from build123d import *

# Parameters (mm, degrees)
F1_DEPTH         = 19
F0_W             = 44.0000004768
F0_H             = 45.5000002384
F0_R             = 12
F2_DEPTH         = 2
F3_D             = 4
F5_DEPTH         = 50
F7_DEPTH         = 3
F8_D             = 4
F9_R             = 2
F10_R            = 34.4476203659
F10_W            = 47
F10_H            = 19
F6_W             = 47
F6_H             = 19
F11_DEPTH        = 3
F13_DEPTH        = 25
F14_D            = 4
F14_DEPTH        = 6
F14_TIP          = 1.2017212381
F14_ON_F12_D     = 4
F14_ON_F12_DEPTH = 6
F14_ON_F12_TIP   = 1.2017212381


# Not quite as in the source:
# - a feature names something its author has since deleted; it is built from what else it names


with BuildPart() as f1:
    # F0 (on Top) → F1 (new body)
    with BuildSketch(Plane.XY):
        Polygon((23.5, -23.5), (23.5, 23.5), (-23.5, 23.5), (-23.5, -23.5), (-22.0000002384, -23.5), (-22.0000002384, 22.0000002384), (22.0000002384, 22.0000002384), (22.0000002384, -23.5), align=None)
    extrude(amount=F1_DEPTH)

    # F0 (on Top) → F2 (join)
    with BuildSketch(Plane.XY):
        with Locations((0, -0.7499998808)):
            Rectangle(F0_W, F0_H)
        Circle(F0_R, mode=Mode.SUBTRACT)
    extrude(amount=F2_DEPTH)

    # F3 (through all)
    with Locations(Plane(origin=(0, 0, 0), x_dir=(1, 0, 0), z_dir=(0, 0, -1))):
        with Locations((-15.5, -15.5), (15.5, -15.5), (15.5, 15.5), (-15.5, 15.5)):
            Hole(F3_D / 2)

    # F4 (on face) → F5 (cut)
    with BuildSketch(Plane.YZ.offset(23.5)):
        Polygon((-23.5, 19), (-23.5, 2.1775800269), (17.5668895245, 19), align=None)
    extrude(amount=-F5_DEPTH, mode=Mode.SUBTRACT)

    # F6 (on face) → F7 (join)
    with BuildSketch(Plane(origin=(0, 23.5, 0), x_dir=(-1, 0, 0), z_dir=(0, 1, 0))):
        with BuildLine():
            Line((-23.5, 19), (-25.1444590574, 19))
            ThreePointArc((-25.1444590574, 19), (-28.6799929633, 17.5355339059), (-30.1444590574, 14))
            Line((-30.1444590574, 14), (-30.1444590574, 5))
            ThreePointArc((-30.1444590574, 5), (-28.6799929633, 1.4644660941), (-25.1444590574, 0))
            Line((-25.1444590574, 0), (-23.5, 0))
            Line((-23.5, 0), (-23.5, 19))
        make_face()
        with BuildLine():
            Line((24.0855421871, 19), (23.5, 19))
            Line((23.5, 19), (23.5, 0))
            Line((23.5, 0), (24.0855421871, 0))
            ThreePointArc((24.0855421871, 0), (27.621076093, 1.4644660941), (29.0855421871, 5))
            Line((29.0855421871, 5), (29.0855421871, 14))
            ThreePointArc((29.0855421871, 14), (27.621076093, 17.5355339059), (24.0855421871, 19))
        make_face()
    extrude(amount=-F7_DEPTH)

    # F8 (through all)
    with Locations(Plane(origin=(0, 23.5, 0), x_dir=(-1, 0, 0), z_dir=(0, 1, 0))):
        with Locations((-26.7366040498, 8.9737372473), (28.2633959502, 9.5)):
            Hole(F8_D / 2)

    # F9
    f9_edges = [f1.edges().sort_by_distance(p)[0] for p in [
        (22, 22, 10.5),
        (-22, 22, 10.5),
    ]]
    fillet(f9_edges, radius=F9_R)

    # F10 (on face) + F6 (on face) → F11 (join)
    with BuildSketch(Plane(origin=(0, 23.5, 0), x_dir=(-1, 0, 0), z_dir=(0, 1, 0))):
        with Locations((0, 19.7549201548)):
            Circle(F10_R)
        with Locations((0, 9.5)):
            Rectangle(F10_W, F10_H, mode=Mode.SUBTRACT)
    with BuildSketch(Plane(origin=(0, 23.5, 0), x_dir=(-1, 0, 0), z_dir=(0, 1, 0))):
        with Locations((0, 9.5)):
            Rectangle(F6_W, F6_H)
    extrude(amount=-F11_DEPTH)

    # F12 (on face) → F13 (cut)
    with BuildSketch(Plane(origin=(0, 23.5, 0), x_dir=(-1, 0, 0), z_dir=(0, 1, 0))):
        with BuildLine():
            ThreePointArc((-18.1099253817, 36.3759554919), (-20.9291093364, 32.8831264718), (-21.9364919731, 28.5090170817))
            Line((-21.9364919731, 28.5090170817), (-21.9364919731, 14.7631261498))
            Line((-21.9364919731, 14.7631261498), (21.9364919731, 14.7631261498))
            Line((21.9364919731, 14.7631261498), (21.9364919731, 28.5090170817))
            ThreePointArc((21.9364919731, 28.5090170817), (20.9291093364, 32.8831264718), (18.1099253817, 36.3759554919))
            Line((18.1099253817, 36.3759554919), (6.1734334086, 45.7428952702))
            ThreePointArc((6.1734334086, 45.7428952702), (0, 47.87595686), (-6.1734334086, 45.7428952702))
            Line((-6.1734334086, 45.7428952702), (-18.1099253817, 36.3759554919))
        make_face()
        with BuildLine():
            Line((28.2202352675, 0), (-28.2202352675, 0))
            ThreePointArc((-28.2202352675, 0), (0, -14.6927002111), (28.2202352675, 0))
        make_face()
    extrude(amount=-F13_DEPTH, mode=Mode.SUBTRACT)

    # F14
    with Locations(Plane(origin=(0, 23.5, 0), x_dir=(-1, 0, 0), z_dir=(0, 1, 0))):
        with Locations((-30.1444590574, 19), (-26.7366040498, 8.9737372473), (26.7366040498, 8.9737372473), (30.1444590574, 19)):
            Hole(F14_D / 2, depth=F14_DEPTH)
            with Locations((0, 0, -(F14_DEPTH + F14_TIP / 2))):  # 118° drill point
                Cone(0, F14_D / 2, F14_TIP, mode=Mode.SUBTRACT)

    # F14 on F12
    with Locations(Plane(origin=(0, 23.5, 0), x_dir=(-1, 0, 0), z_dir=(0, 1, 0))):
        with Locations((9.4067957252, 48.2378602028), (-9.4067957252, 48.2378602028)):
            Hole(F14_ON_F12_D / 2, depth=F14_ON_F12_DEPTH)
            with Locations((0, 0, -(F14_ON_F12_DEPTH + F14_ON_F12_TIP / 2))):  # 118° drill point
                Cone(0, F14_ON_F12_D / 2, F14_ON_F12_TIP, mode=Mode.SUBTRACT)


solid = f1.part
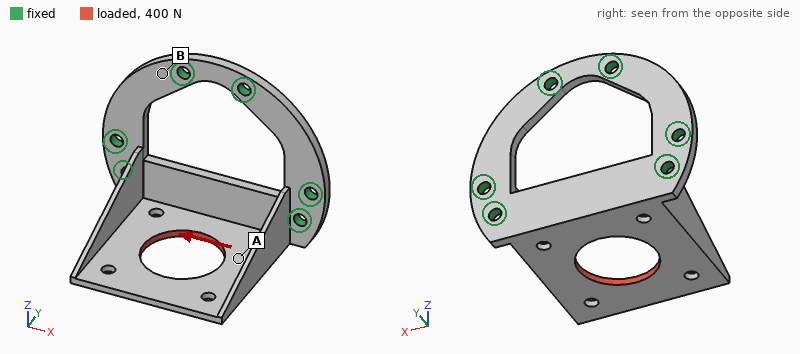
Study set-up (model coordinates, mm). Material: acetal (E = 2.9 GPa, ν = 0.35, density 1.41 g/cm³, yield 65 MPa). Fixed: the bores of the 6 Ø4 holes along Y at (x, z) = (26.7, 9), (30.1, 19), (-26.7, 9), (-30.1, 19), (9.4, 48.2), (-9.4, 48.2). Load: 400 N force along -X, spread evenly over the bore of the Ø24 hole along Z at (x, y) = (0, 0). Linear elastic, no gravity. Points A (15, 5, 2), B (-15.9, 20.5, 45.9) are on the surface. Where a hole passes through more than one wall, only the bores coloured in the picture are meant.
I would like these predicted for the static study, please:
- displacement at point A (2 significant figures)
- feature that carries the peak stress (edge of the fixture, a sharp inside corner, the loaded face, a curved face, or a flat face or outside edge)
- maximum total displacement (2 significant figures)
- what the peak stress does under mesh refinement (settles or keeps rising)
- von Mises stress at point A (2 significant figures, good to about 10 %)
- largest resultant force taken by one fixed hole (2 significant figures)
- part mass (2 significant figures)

0.34 mm
edge of the fixture
1.0 mm
keeps rising
12 MPa
300 N
14 g
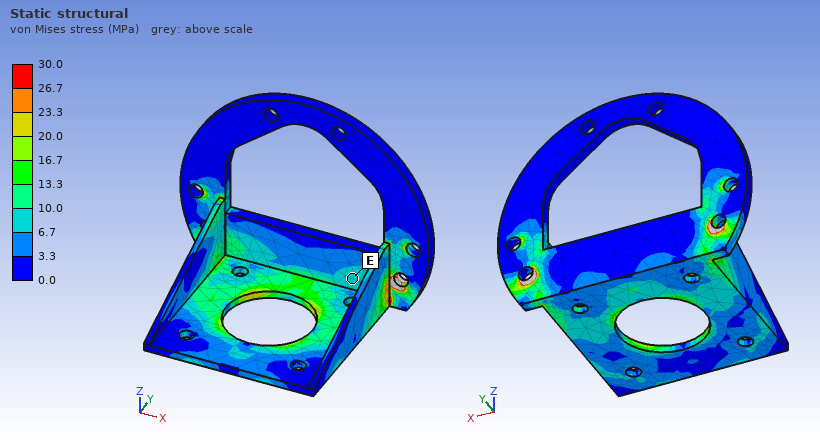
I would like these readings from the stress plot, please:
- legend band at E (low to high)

6.7 to 10.0 MPa
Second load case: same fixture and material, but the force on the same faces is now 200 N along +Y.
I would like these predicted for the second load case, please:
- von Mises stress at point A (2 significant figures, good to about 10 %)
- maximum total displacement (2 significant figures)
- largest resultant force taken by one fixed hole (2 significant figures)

2.9 MPa
0.60 mm
140 N
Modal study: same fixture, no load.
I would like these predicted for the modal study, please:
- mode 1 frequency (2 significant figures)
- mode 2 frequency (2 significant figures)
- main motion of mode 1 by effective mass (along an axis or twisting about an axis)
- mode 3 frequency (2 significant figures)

640 Hz
1100 Hz
along Z
1700 Hz
